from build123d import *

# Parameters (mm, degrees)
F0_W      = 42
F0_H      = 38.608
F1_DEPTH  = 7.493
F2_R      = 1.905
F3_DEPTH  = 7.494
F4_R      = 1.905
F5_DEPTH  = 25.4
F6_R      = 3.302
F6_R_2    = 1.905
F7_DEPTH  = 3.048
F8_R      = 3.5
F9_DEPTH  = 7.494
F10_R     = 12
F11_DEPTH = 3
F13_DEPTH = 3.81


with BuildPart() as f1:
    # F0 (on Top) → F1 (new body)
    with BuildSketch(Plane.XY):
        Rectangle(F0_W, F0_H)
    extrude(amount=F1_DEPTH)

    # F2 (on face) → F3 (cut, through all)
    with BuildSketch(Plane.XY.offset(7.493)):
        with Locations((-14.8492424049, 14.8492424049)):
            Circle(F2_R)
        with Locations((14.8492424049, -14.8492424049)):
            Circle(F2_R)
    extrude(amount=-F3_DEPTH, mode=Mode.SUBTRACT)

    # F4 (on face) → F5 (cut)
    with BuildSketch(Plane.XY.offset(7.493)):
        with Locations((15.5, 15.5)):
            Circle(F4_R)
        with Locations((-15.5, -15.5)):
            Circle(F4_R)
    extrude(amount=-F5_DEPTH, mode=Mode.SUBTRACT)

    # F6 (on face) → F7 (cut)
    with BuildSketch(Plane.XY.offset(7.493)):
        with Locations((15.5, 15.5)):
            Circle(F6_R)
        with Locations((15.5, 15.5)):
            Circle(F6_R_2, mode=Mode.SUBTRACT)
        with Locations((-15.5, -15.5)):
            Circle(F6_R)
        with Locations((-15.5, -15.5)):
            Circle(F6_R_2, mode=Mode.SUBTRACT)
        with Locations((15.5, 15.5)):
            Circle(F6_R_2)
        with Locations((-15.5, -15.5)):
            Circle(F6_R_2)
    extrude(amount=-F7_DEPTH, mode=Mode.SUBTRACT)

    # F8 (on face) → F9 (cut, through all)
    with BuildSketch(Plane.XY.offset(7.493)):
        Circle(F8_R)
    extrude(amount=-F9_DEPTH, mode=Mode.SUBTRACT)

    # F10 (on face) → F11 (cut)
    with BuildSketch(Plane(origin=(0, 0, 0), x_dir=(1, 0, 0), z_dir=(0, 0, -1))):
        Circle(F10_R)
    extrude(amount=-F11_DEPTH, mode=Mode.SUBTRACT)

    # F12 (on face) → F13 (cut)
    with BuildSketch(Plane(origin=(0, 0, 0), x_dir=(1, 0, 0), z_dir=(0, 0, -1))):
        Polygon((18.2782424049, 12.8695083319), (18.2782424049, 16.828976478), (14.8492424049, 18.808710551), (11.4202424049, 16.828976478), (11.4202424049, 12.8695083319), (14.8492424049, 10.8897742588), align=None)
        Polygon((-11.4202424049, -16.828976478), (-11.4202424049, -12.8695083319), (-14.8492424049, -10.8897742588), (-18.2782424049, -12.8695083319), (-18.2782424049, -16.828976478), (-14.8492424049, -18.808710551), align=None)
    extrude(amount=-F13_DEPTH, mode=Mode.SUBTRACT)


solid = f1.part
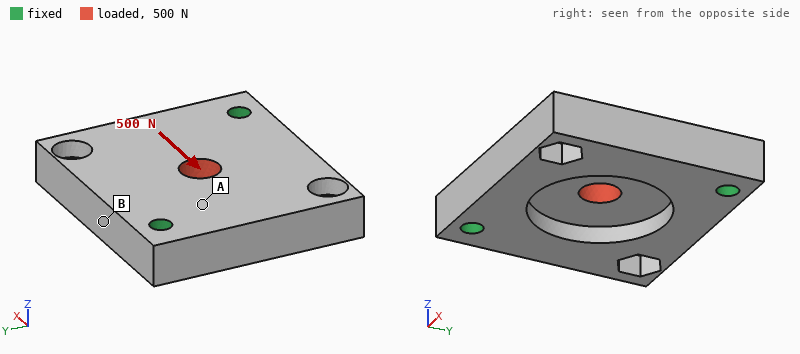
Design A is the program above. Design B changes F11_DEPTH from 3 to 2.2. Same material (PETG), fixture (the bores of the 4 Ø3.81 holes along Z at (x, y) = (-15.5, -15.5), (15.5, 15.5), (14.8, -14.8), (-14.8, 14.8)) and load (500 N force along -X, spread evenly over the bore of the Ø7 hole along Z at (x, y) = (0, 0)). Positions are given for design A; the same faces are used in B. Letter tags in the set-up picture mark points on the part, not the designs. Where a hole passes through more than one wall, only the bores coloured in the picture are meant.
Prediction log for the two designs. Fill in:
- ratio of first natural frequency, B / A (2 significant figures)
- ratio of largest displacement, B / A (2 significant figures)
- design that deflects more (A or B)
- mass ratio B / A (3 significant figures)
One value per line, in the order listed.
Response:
0.99
0.90
A
1.03
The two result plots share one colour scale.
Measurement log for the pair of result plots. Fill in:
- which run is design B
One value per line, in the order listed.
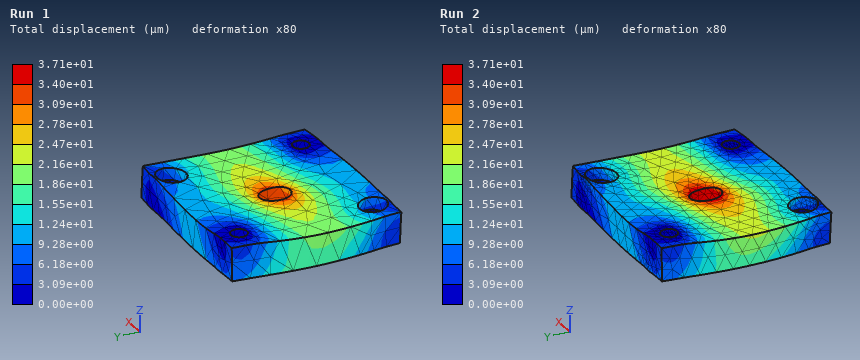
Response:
Run 1
